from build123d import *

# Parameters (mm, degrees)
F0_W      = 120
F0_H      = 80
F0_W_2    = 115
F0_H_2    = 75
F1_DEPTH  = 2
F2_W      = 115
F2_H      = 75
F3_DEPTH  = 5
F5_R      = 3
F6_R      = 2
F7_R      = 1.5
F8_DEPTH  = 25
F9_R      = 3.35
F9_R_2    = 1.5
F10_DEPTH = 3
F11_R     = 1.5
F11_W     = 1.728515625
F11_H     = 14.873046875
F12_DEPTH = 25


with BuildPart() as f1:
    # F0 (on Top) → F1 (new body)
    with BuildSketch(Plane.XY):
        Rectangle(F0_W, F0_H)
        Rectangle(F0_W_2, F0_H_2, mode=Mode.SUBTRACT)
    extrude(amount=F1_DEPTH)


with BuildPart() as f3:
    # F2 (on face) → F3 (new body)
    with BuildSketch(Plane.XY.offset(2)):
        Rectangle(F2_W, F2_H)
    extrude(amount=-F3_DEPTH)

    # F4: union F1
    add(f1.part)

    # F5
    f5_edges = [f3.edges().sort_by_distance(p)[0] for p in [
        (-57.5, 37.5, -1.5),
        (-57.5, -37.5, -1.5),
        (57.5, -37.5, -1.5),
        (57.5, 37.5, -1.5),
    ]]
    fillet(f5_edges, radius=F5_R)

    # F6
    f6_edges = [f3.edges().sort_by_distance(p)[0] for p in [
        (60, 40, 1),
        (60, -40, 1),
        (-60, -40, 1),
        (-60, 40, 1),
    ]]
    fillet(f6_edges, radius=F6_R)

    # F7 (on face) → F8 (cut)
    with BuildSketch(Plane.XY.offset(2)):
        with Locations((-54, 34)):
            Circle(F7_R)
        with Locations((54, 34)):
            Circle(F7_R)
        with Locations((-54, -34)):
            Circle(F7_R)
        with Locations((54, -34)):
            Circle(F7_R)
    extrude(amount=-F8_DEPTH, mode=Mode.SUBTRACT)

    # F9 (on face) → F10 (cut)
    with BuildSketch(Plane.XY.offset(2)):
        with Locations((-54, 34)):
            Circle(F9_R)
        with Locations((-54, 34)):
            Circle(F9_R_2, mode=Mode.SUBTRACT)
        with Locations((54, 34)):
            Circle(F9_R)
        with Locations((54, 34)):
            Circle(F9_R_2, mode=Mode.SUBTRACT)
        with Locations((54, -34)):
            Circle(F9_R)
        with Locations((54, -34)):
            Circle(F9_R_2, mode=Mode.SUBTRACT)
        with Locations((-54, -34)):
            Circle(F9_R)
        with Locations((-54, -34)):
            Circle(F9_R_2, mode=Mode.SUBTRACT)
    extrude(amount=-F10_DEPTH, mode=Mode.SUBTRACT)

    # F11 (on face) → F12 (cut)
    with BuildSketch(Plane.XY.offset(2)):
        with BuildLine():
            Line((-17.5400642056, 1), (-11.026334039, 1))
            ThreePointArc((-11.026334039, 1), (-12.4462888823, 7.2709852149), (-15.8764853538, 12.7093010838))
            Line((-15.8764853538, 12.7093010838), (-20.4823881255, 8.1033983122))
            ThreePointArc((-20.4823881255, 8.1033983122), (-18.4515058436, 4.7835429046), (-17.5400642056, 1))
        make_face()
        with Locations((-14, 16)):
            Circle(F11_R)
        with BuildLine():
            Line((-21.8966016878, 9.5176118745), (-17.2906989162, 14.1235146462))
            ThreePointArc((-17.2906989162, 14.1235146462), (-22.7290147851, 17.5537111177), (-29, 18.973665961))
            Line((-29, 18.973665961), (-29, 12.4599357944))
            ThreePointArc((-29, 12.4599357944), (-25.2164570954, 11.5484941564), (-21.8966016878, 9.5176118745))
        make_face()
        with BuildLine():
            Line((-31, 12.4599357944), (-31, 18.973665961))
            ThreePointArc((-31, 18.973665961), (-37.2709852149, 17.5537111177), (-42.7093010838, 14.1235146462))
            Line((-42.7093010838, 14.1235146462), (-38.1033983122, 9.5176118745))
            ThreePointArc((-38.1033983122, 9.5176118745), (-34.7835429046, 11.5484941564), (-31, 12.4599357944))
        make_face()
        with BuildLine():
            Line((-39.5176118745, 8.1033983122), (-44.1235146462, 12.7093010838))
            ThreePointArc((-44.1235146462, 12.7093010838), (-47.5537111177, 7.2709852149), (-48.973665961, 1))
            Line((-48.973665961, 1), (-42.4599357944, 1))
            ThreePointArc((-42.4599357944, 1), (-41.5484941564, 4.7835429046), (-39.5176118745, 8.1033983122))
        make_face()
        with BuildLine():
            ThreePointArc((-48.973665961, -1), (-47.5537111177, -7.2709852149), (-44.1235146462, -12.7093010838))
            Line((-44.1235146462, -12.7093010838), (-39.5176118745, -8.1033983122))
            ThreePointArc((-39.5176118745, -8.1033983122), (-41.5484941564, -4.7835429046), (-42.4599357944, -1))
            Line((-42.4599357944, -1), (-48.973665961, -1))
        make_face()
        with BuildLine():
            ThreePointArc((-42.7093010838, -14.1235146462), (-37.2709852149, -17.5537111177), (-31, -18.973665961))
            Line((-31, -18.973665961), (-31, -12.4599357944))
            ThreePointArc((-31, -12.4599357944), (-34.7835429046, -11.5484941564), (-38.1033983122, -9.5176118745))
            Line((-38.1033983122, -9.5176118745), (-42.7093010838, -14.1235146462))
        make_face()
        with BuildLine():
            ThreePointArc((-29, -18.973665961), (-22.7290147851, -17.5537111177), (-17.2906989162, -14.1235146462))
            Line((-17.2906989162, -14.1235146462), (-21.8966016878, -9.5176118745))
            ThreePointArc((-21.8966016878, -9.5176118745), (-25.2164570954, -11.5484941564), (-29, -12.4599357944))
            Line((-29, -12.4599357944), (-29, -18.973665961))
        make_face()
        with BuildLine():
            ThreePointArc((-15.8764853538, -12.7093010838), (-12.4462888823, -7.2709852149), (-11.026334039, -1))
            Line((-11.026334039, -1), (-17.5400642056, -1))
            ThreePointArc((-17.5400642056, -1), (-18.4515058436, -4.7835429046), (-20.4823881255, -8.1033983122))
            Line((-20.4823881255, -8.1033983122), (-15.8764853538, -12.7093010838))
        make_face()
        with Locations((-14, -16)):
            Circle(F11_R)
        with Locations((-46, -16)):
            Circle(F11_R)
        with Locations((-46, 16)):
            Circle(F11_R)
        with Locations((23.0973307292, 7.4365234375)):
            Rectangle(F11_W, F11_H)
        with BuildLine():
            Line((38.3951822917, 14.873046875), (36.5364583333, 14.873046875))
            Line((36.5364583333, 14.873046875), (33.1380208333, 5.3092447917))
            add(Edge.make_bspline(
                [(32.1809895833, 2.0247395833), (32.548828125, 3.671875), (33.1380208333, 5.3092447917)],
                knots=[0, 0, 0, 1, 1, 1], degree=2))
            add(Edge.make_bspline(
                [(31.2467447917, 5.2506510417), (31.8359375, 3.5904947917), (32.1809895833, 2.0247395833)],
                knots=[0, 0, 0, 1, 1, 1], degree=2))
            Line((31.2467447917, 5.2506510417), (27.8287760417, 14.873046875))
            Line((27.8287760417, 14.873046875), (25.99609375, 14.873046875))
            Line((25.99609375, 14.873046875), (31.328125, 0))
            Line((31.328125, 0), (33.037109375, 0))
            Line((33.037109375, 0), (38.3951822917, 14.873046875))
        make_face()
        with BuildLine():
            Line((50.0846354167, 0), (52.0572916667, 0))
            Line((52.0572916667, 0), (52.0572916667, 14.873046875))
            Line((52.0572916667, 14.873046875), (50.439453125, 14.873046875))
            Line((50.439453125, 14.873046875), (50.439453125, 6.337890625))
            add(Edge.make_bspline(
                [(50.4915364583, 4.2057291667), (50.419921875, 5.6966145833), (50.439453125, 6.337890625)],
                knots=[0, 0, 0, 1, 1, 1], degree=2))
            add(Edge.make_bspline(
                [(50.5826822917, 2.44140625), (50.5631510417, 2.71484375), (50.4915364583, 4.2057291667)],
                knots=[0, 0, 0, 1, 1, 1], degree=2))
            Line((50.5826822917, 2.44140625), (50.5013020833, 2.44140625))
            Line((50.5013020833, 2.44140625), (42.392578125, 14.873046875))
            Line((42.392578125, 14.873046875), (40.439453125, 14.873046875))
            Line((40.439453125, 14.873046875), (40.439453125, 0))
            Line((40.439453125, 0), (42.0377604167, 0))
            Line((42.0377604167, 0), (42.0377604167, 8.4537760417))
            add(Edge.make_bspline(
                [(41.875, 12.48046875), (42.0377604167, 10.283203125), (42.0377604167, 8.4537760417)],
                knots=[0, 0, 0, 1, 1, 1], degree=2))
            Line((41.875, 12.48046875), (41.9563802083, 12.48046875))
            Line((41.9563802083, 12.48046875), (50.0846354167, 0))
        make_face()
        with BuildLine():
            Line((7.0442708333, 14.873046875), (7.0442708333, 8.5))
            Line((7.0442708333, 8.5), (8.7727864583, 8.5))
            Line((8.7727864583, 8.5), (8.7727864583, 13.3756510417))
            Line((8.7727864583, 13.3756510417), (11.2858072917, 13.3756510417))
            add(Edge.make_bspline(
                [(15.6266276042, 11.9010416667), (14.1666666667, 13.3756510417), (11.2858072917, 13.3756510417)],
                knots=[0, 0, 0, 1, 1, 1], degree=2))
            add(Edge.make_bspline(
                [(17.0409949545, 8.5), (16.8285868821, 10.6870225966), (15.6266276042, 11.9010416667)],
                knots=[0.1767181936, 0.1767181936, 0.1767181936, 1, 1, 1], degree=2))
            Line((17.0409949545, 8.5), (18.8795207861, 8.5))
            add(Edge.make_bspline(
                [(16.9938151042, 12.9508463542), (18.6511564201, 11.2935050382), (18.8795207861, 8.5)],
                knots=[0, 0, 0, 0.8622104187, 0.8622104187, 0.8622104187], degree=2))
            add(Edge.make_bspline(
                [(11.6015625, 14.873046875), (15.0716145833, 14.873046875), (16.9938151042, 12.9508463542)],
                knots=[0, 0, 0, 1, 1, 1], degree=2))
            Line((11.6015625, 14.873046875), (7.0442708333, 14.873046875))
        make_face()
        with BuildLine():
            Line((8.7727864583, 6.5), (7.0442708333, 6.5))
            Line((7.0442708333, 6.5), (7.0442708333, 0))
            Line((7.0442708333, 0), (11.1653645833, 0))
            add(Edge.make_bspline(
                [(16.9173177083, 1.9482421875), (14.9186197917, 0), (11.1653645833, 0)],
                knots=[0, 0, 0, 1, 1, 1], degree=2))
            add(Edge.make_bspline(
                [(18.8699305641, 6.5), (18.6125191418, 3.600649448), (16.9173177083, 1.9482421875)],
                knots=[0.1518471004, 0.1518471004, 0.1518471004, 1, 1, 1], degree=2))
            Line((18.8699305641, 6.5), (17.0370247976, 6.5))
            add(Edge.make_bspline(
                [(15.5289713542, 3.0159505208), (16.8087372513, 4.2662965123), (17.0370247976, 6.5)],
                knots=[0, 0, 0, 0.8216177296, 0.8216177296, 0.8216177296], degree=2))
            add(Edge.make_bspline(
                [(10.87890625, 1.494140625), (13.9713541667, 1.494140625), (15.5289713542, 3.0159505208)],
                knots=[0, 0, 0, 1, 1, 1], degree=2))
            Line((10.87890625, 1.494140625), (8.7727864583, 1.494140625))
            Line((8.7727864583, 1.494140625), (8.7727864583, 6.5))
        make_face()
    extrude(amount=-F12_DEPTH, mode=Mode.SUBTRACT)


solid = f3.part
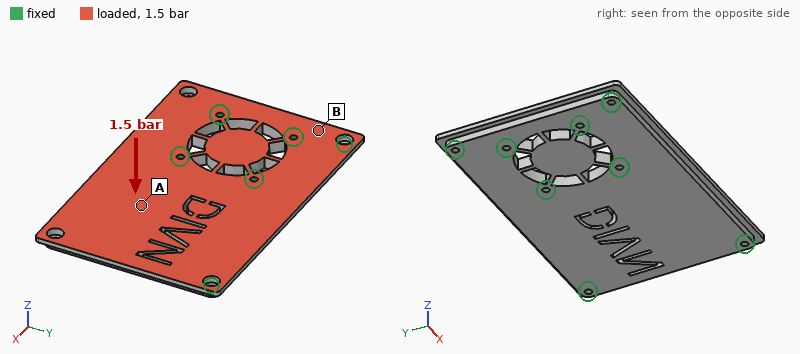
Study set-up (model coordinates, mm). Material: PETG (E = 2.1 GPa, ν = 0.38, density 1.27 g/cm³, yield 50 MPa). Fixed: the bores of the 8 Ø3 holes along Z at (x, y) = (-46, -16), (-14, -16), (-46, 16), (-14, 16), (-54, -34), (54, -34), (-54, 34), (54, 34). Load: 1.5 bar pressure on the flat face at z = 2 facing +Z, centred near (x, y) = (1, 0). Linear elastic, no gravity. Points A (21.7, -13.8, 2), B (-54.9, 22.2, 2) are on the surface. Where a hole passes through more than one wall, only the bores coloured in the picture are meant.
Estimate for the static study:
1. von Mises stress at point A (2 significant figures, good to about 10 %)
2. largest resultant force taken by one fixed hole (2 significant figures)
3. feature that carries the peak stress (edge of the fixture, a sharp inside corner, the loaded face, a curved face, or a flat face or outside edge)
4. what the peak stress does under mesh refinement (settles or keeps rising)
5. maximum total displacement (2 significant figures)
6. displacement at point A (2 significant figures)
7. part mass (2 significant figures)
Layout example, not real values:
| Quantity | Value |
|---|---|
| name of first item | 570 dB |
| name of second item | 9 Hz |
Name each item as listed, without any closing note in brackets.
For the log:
| Quantity | Value |
|---|---|
| von Mises stress at point A | 11 MPa |
| largest resultant force taken by one fixed hole | 350 N |
| feature that carries the peak stress | edge of the fixture |
| what the peak stress does under mesh refinement | keeps rising |
| maximum total displacement | 1.7 mm |
| displacement at point A | 1.0 mm |
| part mass | 52 g |
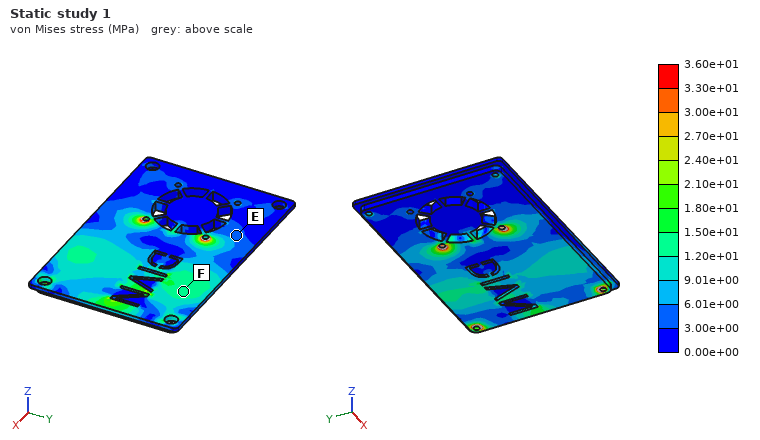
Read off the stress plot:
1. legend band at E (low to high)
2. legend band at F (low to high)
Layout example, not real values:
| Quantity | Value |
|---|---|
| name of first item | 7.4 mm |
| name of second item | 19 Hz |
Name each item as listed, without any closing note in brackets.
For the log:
| Quantity | Value |
|---|---|
| legend band at E | 3.00e+00 to 6.01e+00 MPa |
| legend band at F | 1.20e+01 to 1.50e+01 MPa |
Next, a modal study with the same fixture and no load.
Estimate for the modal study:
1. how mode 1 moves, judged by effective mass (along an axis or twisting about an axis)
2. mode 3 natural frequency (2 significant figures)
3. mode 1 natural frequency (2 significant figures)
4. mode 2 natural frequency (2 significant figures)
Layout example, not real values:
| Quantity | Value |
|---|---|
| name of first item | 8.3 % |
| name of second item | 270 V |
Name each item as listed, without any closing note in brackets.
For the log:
| Quantity | Value |
|---|---|
| how mode 1 moves, judged by effective mass | along Z |
| mode 3 natural frequency | 1100 Hz |
| mode 1 natural frequency | 800 Hz |
| mode 2 natural frequency | 1100 Hz |
